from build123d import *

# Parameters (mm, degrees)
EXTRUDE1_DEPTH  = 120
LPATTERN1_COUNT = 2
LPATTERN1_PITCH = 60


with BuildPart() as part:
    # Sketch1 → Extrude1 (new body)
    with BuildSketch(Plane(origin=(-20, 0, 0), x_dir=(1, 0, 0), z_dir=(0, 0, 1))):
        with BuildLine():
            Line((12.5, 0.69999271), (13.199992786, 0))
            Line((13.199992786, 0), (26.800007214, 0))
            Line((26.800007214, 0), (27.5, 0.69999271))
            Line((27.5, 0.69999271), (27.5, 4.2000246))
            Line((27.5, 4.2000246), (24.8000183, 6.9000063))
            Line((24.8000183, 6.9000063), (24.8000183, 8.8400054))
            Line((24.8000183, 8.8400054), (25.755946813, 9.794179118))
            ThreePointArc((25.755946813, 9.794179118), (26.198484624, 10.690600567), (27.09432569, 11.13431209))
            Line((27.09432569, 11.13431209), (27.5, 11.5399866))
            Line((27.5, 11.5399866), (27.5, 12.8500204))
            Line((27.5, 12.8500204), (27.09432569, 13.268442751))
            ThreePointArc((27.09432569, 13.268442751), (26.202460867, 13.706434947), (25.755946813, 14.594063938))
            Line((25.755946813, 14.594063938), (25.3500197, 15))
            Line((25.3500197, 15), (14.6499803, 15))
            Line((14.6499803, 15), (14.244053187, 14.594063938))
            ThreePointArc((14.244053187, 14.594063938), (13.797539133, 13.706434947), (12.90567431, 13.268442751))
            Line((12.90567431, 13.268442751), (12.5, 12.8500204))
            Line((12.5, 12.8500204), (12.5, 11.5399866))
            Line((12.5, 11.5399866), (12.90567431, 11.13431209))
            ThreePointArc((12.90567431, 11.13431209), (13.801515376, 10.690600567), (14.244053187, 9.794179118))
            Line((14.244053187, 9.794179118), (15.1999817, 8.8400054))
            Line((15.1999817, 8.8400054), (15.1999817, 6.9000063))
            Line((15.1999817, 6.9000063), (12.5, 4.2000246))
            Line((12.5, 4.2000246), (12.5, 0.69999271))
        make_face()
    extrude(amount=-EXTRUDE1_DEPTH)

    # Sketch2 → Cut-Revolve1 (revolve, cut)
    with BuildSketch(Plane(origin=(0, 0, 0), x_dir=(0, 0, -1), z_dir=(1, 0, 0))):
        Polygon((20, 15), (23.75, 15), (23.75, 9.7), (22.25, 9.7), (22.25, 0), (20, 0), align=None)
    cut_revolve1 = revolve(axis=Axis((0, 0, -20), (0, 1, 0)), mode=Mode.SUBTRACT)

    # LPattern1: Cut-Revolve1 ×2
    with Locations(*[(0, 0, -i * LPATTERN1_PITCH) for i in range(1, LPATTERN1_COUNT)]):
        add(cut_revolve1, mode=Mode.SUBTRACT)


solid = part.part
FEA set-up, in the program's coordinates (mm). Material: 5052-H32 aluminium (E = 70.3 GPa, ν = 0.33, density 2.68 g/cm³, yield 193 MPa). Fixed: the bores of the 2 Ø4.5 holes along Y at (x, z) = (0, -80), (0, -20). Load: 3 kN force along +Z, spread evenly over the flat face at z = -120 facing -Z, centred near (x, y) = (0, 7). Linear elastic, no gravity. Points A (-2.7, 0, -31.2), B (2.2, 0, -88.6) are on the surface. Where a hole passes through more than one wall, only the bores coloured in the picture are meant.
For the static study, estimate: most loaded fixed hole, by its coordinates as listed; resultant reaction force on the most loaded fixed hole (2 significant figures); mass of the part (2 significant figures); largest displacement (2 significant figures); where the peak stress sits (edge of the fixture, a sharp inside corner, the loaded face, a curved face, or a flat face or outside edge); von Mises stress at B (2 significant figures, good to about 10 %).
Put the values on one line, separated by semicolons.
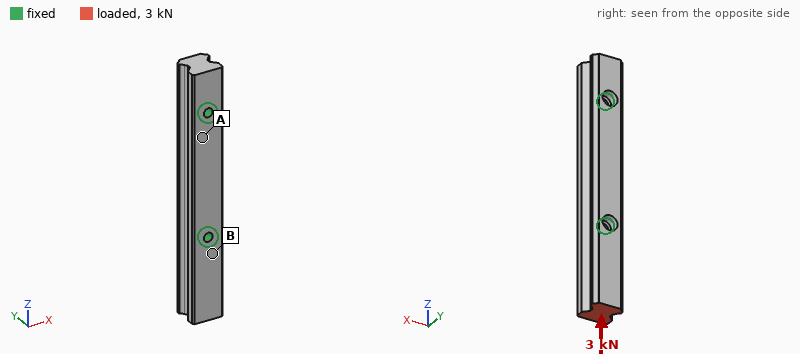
(0, -80); 2.8 kN; 60 g; 17 µm; edge of the fixture; 14 MPa
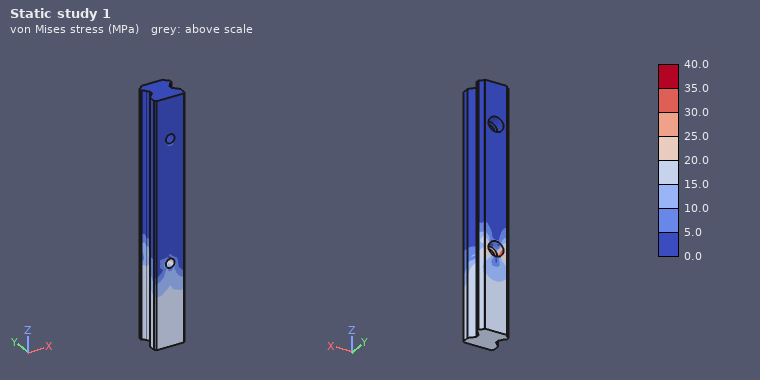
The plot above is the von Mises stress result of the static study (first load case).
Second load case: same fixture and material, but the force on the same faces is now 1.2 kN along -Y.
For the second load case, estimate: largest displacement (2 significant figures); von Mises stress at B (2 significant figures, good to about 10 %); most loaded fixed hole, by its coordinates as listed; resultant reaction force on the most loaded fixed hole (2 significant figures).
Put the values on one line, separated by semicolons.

0.16 mm; 92 MPa; (0, -80); 1.5 kN
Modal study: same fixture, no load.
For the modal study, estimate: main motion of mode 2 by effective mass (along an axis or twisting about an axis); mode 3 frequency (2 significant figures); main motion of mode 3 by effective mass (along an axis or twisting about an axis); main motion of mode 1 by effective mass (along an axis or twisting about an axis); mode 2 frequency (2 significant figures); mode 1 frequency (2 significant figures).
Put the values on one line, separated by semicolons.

along Y; 12 kHz; along X; along X; 5700 Hz; 5100 Hz
